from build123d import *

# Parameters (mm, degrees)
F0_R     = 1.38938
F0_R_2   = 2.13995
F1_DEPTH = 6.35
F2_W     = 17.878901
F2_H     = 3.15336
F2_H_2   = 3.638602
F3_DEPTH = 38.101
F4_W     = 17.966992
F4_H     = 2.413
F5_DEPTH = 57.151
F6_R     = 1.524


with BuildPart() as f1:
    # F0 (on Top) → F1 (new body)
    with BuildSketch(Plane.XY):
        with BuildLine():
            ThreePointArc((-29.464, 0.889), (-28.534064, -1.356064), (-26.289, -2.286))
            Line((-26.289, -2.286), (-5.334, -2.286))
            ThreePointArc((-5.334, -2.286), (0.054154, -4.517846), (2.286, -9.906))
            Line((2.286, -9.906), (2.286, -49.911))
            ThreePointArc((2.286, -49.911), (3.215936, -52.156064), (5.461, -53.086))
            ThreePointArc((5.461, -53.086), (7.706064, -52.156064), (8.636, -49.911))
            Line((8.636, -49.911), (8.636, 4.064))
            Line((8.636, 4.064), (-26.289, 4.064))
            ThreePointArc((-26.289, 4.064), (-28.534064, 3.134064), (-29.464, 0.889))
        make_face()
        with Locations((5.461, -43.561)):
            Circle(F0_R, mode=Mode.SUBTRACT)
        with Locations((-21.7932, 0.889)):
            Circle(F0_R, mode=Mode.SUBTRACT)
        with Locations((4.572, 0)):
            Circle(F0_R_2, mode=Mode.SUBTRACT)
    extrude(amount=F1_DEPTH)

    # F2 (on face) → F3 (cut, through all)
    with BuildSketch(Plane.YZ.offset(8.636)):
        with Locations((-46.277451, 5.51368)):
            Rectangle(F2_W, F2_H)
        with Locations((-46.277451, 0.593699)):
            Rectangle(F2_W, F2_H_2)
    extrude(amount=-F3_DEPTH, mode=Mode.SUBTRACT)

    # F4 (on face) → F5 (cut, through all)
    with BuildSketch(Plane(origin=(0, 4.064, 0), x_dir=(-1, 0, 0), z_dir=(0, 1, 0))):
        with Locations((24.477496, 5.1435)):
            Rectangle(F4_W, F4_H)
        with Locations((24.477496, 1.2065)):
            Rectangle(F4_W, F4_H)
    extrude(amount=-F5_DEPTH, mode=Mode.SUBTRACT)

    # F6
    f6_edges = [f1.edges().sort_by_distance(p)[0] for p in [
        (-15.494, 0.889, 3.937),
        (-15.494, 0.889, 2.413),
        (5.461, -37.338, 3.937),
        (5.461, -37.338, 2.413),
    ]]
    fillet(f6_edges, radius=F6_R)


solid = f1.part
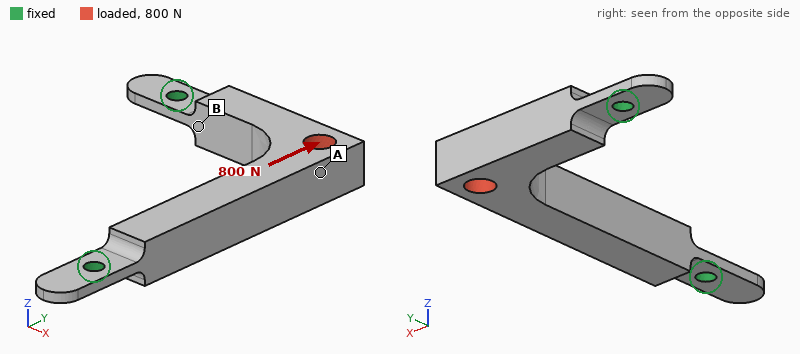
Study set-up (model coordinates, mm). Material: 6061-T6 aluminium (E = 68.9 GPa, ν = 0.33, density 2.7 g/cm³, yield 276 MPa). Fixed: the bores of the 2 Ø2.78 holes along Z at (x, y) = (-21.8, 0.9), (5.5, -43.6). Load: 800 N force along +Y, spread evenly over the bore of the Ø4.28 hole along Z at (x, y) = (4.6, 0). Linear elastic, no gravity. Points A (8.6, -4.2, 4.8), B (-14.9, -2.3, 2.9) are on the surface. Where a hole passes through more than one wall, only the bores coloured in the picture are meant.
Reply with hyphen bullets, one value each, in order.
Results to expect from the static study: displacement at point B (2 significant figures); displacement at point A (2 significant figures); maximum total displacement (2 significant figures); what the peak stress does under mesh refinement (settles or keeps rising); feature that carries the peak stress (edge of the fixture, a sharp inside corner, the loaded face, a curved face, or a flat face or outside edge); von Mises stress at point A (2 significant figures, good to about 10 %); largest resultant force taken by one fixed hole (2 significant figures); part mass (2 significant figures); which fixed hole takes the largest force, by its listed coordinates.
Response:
- 5.4 µm
- 16 µm
- 19 µm
- keeps rising
- edge of the fixture
- 29 MPa
- 760 N
- 7.1 g
- (5.5, -43.6)
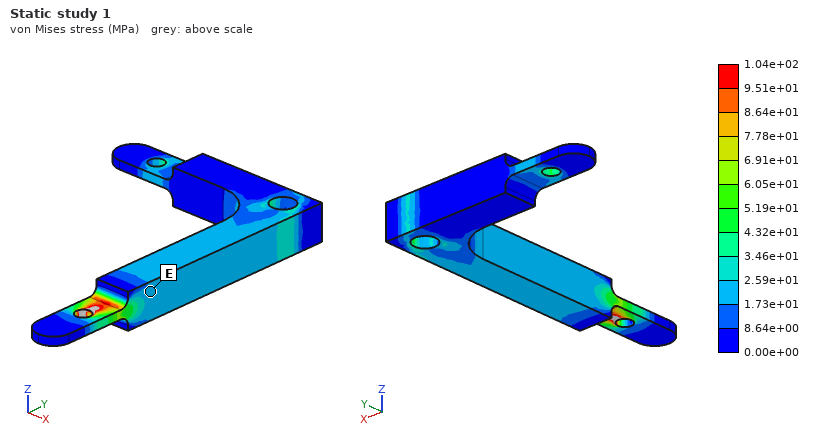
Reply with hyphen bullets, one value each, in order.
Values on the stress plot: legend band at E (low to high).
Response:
- 1.73e+01 to 2.59e+01 MPa
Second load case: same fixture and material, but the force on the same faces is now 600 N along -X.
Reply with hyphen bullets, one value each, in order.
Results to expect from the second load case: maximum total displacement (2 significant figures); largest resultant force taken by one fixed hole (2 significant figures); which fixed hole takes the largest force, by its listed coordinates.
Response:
- 11 µm
- 590 N
- (-21.8, 0.9)
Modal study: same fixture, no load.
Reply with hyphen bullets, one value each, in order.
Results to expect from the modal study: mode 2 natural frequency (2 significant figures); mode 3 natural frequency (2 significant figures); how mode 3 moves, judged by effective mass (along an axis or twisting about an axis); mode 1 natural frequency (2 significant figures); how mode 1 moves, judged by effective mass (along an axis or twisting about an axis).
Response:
- 9000 Hz
- 11 kHz
- along X
- 1300 Hz
- along Z
